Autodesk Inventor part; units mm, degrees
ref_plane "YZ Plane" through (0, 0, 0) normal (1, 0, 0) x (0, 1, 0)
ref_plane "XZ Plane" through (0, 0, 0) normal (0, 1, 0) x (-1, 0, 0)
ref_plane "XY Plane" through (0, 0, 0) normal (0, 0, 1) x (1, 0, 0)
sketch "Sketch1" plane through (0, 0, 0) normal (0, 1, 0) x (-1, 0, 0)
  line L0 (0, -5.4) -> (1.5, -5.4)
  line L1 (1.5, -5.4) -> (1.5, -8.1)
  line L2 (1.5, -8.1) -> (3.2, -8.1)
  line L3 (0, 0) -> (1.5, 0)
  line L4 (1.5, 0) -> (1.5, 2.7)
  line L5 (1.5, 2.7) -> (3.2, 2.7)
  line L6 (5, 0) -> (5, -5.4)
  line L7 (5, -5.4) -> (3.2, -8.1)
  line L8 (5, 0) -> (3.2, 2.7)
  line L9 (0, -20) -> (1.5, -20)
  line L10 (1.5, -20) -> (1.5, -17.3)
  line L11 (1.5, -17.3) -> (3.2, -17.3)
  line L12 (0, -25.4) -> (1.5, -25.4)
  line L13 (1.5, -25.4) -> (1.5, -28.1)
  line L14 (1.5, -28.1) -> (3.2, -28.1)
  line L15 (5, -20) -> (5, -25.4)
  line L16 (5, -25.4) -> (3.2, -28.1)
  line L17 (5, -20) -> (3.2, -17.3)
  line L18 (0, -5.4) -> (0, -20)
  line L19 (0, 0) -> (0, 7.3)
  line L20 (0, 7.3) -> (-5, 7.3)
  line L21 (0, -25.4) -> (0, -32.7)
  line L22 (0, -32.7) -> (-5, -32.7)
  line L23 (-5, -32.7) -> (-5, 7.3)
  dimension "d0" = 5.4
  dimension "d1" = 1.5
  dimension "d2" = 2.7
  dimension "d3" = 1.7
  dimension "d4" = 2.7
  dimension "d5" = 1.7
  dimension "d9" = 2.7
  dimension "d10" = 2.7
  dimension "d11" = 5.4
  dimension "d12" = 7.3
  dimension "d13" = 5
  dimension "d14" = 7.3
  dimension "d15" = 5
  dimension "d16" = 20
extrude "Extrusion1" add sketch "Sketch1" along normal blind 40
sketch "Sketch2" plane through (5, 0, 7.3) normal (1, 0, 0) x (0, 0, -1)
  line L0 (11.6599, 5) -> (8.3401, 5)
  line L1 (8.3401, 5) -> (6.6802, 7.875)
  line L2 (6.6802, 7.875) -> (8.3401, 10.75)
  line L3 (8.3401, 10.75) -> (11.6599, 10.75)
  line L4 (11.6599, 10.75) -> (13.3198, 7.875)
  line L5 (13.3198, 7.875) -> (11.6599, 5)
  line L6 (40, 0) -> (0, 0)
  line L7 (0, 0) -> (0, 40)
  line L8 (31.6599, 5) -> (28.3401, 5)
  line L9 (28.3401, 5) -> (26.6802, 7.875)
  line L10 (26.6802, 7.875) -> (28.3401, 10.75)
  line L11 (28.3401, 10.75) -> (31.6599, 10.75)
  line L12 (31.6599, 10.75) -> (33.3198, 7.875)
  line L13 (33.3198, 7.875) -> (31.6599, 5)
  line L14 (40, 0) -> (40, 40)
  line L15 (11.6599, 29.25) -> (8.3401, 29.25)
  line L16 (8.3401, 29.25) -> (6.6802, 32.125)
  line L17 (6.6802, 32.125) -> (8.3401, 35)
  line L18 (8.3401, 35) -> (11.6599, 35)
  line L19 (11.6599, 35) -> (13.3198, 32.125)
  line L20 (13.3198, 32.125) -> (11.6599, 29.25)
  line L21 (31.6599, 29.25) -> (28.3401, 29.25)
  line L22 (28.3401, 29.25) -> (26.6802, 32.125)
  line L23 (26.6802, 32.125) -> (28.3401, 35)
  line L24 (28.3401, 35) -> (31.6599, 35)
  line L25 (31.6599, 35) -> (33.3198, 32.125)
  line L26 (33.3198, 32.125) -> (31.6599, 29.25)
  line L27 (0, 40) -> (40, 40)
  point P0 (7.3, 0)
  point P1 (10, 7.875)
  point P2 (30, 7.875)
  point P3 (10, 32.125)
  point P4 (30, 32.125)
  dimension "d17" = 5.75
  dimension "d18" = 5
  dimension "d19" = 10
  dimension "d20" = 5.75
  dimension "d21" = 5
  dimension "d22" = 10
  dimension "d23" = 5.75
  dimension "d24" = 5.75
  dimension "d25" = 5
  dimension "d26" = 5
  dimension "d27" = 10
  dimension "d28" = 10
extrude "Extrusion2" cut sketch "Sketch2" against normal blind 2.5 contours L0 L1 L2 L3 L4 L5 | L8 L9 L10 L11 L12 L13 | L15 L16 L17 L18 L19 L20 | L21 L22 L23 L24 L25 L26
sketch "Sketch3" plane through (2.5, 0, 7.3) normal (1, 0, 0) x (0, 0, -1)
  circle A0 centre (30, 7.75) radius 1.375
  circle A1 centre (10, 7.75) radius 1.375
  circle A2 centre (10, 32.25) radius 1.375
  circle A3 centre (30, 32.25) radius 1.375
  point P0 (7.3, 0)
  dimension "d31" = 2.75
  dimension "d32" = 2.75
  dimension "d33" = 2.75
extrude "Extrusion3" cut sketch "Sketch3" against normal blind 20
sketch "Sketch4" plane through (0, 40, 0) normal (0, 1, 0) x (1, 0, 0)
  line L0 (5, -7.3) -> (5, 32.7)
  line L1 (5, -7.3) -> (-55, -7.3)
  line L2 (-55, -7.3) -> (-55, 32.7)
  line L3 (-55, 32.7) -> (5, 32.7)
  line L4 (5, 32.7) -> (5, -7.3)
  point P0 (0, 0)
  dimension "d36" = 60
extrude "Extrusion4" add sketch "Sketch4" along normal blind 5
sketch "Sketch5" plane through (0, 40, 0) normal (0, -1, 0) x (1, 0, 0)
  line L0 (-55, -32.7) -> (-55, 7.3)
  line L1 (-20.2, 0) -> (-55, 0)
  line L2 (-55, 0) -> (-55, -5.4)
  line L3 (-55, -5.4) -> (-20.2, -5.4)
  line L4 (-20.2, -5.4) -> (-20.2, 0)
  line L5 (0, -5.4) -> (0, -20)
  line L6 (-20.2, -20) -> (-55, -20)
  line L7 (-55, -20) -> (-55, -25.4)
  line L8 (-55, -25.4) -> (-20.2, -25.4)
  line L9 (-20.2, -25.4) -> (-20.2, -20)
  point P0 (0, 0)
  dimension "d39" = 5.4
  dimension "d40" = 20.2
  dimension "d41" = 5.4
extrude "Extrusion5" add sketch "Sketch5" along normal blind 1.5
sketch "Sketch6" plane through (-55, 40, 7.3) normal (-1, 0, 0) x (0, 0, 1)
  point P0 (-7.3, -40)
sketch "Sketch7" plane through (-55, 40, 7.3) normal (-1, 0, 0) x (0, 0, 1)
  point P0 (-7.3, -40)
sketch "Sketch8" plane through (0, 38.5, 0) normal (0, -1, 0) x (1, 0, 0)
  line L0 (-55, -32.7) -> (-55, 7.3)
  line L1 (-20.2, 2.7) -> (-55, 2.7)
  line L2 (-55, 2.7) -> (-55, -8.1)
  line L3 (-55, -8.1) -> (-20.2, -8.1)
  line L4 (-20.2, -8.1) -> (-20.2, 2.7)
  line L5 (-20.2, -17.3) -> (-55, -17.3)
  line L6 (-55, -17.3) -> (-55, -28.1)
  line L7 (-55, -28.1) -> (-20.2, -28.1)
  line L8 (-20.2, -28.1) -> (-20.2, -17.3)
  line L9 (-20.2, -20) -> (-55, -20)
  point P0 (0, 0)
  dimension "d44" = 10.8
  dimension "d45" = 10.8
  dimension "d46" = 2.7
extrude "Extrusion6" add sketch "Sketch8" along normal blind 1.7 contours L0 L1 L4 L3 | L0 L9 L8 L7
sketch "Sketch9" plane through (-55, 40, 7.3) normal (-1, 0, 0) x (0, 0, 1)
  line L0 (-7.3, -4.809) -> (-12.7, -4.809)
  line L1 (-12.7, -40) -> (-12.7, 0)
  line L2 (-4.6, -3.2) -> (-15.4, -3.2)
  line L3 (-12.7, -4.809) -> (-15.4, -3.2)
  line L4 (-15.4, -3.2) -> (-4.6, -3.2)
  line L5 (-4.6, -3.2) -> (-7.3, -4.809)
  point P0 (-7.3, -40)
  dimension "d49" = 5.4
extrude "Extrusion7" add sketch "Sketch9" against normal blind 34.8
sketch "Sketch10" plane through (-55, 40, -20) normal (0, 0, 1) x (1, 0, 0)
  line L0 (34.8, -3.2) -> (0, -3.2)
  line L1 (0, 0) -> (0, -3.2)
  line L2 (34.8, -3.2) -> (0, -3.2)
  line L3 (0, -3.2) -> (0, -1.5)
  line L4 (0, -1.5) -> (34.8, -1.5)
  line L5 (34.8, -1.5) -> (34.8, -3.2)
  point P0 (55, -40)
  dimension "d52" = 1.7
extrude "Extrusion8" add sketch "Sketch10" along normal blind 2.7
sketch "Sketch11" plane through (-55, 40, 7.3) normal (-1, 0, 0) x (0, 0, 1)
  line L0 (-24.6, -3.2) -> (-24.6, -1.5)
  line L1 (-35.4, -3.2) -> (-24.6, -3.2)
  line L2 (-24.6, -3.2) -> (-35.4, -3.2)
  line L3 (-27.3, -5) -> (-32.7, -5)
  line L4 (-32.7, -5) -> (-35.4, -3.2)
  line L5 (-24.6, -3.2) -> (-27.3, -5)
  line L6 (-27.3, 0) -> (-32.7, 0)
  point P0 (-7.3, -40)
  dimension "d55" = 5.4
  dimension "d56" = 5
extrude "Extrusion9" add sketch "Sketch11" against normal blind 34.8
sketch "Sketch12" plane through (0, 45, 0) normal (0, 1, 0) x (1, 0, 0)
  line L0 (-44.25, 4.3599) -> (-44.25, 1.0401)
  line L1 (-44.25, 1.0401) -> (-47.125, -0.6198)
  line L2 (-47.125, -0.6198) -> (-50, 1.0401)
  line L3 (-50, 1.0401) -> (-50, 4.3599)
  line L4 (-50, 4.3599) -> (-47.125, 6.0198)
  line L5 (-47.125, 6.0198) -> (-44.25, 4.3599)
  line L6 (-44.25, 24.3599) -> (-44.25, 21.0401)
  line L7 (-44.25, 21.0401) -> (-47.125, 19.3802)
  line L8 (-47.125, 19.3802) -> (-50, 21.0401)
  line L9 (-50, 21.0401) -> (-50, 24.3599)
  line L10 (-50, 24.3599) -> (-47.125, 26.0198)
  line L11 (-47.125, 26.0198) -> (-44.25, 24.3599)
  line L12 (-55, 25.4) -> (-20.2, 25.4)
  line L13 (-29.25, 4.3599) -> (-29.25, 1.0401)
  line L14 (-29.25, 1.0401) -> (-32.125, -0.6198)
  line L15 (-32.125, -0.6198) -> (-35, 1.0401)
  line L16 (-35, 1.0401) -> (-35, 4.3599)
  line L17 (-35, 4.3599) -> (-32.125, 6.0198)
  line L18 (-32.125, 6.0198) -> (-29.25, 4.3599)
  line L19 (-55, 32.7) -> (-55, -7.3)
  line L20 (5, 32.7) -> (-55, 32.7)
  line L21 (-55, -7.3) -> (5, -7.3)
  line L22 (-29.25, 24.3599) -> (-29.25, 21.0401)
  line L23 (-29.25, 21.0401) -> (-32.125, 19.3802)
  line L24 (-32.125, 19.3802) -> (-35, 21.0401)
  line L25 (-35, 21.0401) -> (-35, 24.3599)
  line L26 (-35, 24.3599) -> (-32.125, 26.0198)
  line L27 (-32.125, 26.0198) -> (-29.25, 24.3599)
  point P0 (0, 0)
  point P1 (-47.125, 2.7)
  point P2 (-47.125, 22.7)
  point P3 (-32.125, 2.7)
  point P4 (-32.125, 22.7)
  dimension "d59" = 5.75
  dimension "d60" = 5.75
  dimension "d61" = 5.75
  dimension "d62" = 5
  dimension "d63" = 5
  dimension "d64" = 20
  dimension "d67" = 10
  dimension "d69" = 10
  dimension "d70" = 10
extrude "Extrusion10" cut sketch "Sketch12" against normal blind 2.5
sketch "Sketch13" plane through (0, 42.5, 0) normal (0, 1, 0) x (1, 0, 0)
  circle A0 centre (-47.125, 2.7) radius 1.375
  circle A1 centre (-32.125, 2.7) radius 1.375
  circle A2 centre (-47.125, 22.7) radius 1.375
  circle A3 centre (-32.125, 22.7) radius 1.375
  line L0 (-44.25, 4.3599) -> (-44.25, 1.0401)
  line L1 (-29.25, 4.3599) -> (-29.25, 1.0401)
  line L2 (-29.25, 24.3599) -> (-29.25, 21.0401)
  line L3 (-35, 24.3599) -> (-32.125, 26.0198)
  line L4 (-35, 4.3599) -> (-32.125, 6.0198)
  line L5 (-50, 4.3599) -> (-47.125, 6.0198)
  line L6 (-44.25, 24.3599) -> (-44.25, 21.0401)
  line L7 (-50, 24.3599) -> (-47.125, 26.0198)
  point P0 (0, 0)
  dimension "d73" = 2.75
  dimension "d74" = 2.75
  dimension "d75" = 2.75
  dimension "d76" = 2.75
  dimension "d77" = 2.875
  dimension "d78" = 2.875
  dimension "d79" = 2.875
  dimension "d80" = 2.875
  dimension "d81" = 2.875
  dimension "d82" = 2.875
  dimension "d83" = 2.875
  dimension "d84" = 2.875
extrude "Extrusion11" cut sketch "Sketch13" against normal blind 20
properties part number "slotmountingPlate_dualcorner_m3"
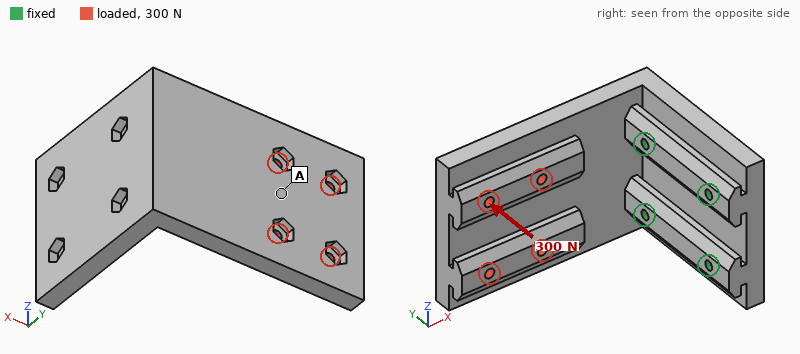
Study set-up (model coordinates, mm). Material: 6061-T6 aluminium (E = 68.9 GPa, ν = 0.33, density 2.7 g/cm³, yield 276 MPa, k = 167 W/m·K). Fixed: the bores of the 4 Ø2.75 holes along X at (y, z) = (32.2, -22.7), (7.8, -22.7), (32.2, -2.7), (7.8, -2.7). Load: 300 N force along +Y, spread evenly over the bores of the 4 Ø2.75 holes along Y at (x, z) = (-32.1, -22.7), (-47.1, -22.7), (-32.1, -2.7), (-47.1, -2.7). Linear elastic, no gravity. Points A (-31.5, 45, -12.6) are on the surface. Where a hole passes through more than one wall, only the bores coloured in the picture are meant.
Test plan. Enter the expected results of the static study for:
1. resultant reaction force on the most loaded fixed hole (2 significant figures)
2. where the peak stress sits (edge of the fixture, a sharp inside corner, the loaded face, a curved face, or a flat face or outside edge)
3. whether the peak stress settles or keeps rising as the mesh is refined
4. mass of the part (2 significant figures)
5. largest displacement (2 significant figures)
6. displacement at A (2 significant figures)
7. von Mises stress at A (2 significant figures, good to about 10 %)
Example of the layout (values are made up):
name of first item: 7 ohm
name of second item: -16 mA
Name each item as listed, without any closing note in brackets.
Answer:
resultant reaction force on the most loaded fixed hole: 380 N
where the peak stress sits: edge of the fixture
whether the peak stress settles or keeps rising as the mesh is refined: keeps rising
mass of the part: 68 g
largest displacement: 0.33 mm
displacement at A: 0.16 mm
von Mises stress at A: 6.7 MPa
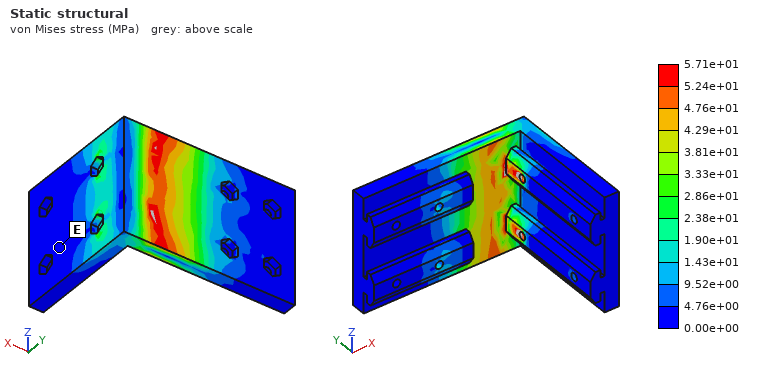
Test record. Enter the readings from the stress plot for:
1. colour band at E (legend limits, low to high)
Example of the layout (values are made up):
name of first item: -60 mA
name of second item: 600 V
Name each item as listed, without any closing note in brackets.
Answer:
colour band at E: 0.00e+00 to 4.76e+00 MPa
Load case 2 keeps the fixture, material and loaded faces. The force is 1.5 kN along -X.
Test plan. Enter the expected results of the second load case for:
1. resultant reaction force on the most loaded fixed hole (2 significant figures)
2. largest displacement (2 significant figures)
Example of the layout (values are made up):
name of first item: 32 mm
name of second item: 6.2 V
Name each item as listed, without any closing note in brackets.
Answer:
resultant reaction force on the most loaded fixed hole: 840 N
largest displacement: 0.16 mm
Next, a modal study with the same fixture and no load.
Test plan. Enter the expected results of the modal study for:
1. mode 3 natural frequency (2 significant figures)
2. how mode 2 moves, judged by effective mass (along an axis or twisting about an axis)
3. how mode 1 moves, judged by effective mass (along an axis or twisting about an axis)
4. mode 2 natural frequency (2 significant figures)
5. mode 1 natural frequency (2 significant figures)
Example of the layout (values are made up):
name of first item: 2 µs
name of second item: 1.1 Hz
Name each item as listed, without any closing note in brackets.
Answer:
mode 3 natural frequency: 4100 Hz
how mode 2 moves, judged by effective mass: along Z
how mode 1 moves, judged by effective mass: along Y
mode 2 natural frequency: 3100 Hz
mode 1 natural frequency: 1200 Hz
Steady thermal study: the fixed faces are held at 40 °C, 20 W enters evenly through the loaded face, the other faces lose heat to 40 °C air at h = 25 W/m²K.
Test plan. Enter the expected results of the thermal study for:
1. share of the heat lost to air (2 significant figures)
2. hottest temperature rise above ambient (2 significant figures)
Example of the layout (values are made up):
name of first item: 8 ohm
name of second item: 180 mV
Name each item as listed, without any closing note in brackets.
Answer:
share of the heat lost to air: 15 %
hottest temperature rise above ambient: 24 K
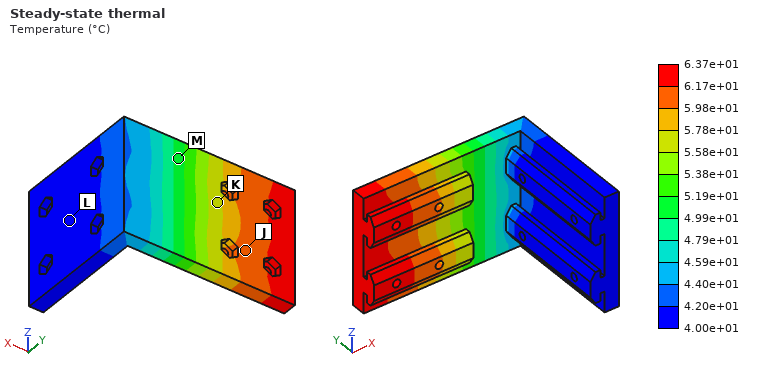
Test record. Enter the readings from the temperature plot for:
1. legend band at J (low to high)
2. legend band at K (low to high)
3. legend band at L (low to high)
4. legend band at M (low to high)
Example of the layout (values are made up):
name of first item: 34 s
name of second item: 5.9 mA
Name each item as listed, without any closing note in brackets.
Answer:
legend band at J: 5.98e+01 to 6.17e+01 °C
legend band at K: 5.58e+01 to 5.78e+01 °C
legend band at L: 4.00e+01 to 4.20e+01 °C
legend band at M: 4.99e+01 to 5.19e+01 °C
